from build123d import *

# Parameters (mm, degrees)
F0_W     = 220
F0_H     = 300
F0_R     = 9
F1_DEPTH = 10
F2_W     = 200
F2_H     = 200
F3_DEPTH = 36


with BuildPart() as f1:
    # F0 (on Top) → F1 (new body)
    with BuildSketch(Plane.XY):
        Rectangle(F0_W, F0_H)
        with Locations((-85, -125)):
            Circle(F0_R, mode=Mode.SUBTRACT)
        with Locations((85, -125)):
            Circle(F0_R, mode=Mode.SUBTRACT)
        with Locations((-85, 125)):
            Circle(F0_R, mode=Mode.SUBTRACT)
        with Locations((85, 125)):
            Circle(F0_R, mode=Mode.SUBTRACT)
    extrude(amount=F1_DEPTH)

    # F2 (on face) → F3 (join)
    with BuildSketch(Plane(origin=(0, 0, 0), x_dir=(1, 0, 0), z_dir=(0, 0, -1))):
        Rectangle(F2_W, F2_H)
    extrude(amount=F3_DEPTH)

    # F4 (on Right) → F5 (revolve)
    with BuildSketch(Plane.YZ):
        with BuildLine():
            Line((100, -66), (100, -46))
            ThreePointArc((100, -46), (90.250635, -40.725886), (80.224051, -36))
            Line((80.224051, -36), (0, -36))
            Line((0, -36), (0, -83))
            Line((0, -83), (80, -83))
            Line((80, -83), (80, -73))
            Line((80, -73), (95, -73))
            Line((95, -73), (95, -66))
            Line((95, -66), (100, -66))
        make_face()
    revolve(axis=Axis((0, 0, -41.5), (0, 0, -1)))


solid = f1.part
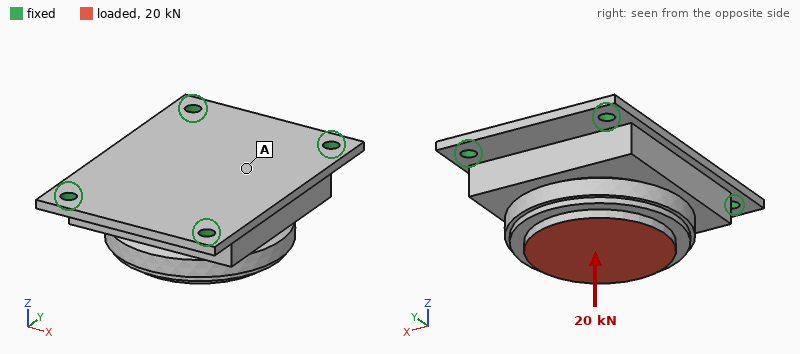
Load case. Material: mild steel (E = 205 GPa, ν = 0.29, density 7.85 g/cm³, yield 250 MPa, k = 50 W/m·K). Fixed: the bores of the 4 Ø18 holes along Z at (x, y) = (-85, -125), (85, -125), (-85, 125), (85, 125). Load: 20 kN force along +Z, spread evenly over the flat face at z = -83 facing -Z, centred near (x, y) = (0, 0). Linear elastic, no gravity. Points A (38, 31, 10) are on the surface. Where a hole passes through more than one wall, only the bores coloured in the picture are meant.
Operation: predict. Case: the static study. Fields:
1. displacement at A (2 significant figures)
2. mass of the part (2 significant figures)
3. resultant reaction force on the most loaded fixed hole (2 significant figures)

16 µm
27 kg
6.5 kN
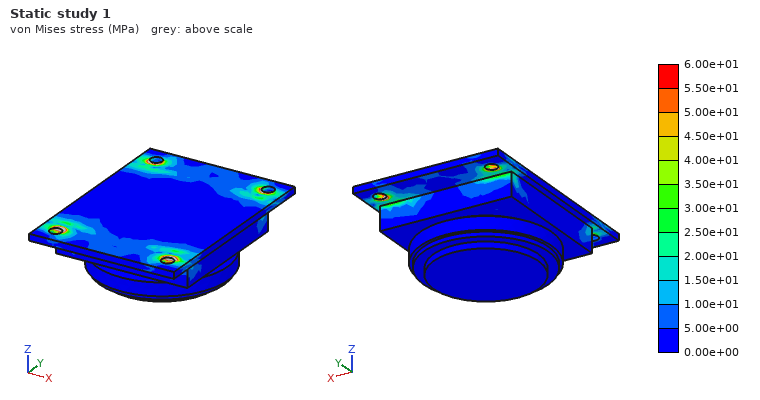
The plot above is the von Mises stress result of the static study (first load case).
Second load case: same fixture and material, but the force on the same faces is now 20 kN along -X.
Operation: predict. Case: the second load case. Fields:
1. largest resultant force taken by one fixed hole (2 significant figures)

8.9 kN
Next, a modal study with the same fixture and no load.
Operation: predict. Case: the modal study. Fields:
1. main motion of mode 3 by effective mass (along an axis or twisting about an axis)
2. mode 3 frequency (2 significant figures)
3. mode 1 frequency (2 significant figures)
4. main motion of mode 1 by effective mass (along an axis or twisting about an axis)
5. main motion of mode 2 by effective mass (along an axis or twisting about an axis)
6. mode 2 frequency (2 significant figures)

along Y
1800 Hz
1200 Hz
along Z
along X
1400 Hz
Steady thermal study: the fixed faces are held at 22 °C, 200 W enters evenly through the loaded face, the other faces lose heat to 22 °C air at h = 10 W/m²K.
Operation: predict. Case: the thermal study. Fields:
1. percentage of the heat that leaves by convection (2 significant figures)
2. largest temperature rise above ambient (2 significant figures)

33 %
53 K
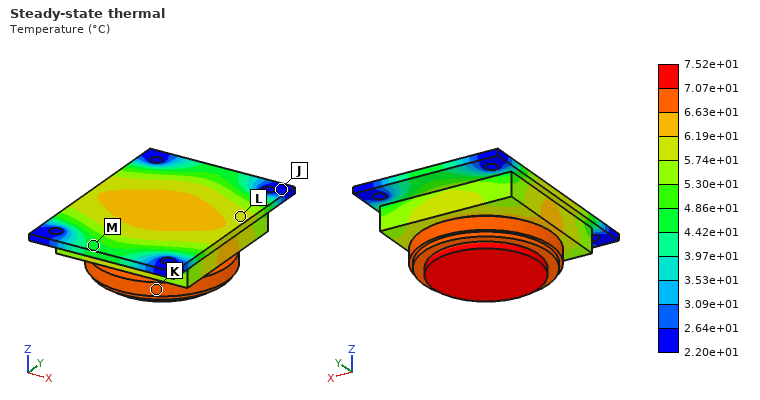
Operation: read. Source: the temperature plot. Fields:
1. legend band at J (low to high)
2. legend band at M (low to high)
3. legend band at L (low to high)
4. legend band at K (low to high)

2.20e+01 to 2.64e+01 °C
4.42e+01 to 4.86e+01 °C
5.74e+01 to 6.19e+01 °C
6.63e+01 to 7.07e+01 °C
